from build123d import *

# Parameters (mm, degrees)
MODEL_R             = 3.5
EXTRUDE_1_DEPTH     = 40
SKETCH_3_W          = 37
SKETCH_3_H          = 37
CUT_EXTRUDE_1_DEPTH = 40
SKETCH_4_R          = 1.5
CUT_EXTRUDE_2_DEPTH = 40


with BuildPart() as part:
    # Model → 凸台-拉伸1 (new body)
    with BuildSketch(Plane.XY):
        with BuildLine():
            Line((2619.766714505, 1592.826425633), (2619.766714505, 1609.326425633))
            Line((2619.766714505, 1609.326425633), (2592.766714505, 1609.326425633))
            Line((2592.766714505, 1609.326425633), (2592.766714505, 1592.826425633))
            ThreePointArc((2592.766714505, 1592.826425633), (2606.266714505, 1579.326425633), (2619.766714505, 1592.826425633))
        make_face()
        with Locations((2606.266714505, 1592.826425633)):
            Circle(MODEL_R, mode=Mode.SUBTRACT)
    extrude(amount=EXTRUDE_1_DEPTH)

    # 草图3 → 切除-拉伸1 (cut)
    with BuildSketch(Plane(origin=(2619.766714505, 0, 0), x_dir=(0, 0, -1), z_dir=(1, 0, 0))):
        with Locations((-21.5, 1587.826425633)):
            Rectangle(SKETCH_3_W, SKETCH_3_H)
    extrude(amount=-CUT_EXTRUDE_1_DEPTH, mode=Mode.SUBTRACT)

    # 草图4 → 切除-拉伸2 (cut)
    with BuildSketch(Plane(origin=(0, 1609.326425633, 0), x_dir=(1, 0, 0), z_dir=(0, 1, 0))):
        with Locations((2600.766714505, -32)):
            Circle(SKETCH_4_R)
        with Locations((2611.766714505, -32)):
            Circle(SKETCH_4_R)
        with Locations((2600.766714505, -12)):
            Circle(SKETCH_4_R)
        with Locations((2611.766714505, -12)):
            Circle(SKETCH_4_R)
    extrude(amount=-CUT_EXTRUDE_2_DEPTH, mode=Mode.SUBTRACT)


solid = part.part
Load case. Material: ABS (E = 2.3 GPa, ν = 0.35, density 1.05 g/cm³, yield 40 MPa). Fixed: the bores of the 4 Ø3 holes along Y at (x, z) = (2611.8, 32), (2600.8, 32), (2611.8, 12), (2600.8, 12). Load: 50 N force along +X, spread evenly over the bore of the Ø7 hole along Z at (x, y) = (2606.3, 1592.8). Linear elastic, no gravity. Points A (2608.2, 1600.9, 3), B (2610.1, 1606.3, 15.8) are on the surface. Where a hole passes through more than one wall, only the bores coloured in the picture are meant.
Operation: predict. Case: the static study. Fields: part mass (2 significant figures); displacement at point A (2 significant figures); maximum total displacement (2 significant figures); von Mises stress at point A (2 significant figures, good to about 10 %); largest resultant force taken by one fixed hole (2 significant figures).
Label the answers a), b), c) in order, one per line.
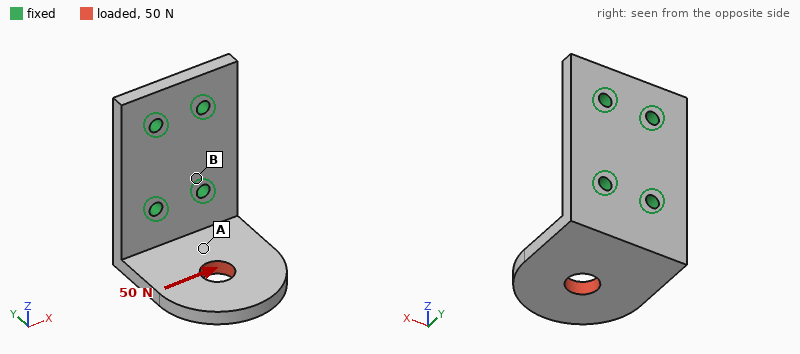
a) 5.2 g
b) 0.13 mm
c) 0.47 mm
d) 4.0 MPa
e) 63 N
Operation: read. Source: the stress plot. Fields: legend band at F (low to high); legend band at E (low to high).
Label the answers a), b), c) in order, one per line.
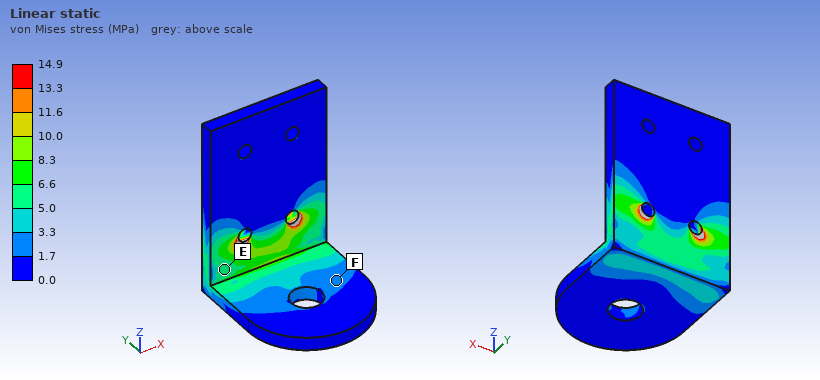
a) 1.7 to 3.3 MPa
b) 5.0 to 6.6 MPa
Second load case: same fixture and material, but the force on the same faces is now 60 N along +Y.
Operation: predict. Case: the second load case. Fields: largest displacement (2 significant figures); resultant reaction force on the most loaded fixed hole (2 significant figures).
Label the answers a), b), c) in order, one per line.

a) 0.66 mm
b) 33 N
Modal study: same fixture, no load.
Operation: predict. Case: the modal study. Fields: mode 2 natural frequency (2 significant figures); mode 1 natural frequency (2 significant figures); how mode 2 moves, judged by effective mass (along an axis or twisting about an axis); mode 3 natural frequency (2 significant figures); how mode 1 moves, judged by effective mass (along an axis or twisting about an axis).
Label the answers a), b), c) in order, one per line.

a) 1400 Hz
b) 690 Hz
c) along X
d) 2600 Hz
e) along Z
